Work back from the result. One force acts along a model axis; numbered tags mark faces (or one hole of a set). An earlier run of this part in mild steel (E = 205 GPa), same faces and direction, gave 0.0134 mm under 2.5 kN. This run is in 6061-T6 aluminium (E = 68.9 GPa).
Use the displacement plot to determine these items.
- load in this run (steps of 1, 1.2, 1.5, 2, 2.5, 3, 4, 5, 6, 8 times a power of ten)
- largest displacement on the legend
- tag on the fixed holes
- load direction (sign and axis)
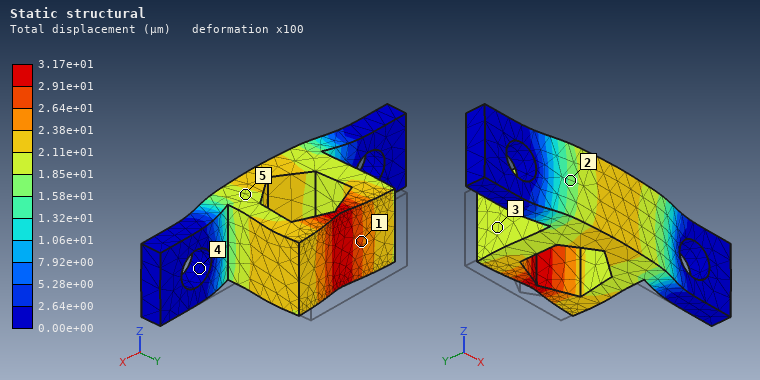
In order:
2 kN
3.17e+01 µm
4
-Y
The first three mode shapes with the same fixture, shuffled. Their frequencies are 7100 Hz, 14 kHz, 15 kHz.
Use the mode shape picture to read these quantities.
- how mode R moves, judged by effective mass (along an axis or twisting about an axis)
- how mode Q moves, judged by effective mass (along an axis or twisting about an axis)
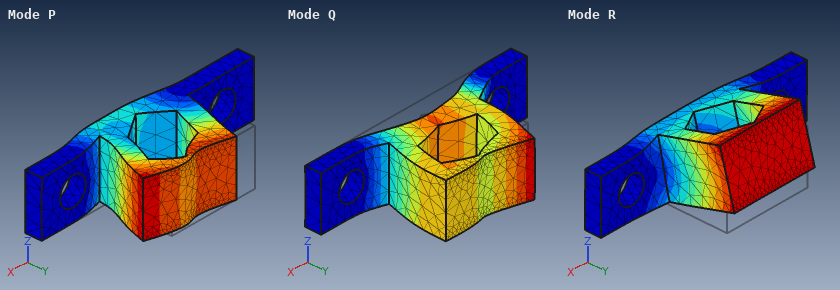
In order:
along Z
along Y
